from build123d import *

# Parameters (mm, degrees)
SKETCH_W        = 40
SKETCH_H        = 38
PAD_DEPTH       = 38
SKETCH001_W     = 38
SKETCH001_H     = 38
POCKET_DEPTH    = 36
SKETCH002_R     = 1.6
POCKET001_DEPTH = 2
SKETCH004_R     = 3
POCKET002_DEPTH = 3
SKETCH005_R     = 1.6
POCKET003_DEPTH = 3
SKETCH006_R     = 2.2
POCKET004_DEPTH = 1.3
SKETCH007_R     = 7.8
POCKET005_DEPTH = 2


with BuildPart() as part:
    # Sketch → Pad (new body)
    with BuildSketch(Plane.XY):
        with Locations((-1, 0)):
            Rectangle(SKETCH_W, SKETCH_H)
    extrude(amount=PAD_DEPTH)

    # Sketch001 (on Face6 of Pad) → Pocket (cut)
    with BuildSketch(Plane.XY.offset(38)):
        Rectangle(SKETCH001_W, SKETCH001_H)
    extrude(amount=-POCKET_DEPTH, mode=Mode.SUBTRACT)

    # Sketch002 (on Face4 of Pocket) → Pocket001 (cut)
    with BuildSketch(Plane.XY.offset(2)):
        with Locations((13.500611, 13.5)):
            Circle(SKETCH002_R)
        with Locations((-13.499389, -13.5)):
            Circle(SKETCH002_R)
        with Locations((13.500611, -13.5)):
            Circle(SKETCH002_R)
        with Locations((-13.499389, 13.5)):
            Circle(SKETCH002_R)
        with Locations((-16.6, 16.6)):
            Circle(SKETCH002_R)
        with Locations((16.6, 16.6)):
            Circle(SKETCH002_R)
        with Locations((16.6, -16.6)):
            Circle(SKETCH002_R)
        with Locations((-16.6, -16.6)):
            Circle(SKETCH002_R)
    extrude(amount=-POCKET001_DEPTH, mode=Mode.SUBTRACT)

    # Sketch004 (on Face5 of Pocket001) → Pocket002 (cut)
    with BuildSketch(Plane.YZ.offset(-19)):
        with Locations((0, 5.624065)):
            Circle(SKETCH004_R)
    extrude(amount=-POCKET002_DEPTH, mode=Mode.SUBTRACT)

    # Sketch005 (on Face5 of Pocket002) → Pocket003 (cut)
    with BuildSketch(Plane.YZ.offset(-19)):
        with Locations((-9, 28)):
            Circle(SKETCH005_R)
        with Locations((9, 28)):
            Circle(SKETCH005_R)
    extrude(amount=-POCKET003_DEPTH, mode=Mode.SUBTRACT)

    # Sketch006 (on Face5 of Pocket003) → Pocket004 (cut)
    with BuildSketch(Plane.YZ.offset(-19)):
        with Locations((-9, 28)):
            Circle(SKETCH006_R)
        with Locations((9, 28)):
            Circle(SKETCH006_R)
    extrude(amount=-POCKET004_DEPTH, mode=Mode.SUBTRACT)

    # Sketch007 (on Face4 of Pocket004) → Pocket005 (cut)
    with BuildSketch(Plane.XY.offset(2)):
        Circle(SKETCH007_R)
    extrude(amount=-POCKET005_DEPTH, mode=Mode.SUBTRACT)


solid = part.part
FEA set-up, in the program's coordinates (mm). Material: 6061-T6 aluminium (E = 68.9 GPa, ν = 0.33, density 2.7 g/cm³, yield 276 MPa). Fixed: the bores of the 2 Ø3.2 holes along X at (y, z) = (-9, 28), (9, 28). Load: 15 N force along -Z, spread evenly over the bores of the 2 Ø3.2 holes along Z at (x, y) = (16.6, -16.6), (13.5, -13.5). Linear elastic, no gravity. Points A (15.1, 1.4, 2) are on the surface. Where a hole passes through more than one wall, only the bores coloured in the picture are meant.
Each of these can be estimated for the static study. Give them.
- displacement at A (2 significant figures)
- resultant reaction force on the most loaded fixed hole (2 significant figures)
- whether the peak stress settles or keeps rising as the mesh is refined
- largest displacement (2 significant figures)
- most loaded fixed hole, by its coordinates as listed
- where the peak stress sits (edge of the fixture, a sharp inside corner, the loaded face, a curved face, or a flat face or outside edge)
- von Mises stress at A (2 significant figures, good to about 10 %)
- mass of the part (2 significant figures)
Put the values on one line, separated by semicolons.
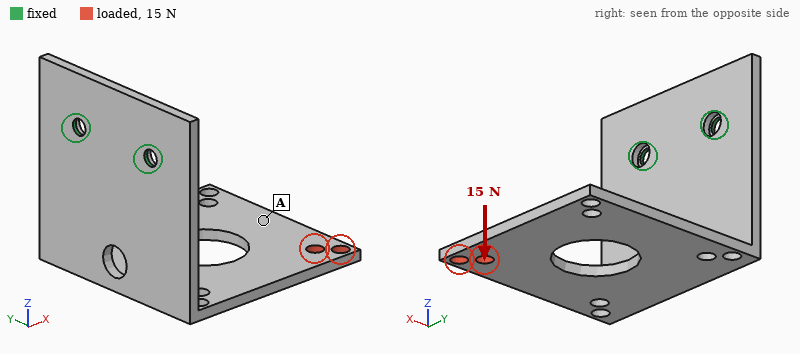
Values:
0.51 mm; 25 N; keeps rising; 0.66 mm; (-9, 28); edge of the fixture; 8.5 MPa; 14 g
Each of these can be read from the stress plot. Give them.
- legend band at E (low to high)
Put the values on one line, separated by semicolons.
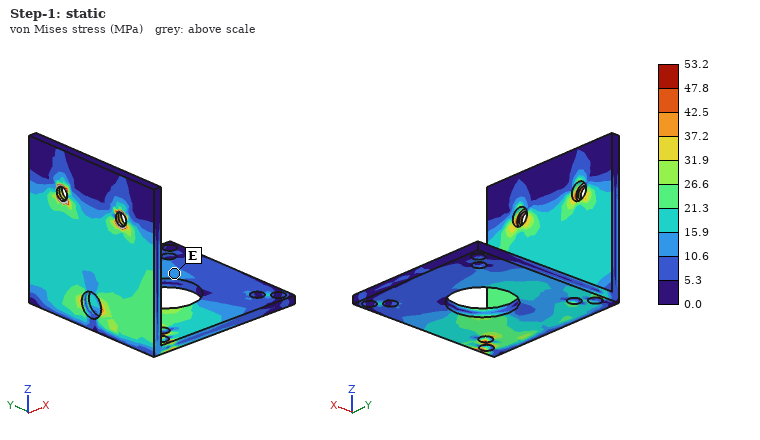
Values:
10.6 to 15.9 MPa
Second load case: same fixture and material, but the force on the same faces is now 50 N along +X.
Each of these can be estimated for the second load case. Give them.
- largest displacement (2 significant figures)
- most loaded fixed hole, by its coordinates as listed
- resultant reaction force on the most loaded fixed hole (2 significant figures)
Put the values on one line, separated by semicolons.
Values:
0.74 mm; (-9, 28); 66 N
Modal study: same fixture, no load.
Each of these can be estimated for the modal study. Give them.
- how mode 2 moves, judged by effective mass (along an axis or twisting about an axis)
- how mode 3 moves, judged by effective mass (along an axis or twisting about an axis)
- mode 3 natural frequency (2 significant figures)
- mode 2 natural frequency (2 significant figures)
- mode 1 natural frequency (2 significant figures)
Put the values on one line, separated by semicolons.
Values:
along Y; along X; 1300 Hz; 880 Hz; 470 Hz
